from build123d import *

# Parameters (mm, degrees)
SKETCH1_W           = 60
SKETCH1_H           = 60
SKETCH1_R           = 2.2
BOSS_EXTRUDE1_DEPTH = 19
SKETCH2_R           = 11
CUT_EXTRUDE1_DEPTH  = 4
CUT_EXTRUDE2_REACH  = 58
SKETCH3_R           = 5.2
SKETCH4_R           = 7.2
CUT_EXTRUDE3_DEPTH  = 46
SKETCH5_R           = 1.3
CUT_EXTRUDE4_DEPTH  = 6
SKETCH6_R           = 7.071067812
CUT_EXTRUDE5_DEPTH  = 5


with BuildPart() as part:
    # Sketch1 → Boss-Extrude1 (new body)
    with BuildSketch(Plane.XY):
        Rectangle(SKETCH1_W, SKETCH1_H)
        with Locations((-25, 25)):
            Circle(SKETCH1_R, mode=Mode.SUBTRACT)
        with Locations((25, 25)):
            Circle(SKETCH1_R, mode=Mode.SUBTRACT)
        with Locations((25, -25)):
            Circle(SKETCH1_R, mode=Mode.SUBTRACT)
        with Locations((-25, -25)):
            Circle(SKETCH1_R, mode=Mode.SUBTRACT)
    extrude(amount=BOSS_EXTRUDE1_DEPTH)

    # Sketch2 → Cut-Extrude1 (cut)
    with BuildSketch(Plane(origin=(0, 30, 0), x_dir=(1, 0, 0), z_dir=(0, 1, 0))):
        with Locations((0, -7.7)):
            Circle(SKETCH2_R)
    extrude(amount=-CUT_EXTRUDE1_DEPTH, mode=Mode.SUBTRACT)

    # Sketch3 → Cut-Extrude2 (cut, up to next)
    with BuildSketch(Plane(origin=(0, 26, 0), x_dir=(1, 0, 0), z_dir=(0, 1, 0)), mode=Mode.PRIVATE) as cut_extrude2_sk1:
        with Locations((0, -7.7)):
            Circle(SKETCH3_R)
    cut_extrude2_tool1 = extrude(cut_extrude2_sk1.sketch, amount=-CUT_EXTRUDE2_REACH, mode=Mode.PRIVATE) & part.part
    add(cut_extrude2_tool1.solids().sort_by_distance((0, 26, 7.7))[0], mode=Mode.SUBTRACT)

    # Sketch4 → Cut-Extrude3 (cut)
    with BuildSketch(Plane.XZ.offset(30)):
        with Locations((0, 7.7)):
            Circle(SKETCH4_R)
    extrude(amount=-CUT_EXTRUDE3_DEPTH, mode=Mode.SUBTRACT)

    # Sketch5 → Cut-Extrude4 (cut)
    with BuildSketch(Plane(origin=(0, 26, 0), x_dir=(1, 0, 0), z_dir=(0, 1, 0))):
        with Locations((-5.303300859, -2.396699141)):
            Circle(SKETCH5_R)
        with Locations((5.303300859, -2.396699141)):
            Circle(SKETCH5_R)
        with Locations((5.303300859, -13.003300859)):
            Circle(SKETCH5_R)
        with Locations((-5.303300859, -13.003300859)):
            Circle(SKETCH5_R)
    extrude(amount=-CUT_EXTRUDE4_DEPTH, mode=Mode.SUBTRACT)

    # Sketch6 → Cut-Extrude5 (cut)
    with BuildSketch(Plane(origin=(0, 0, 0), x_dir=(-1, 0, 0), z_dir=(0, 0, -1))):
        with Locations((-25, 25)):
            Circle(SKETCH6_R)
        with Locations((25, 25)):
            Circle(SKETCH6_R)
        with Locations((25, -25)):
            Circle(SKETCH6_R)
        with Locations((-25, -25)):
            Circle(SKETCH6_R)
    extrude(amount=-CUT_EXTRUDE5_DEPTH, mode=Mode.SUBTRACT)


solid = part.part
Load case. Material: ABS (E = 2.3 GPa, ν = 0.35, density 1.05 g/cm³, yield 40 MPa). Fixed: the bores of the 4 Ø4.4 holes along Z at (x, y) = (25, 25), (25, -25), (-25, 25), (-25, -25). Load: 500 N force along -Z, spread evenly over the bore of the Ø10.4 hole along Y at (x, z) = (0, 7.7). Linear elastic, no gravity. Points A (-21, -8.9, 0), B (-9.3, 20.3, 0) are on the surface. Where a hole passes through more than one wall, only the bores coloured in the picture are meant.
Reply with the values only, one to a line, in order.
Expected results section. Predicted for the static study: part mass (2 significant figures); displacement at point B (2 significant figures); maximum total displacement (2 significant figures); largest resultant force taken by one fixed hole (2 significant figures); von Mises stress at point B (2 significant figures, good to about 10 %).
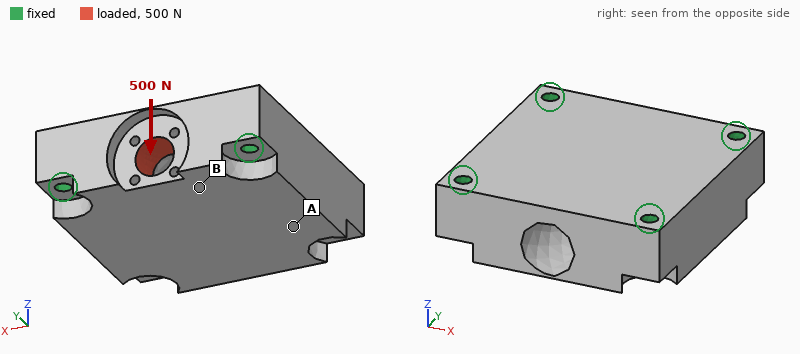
58 g
38 µm
72 µm
230 N
1.5 MPa
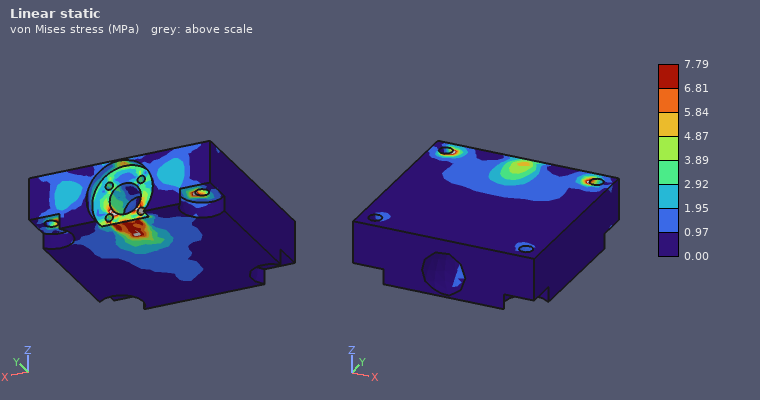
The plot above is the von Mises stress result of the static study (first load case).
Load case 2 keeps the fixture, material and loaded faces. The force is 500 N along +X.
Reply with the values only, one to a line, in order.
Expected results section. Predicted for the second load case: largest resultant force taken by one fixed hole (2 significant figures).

210 N
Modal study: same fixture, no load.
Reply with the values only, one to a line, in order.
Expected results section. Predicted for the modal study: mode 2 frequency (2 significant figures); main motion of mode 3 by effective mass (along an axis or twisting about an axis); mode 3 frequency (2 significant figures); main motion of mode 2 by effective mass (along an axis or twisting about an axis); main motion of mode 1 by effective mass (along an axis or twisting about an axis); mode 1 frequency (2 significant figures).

5900 Hz
along X
6200 Hz
twisting about Y
along Z
4400 Hz
